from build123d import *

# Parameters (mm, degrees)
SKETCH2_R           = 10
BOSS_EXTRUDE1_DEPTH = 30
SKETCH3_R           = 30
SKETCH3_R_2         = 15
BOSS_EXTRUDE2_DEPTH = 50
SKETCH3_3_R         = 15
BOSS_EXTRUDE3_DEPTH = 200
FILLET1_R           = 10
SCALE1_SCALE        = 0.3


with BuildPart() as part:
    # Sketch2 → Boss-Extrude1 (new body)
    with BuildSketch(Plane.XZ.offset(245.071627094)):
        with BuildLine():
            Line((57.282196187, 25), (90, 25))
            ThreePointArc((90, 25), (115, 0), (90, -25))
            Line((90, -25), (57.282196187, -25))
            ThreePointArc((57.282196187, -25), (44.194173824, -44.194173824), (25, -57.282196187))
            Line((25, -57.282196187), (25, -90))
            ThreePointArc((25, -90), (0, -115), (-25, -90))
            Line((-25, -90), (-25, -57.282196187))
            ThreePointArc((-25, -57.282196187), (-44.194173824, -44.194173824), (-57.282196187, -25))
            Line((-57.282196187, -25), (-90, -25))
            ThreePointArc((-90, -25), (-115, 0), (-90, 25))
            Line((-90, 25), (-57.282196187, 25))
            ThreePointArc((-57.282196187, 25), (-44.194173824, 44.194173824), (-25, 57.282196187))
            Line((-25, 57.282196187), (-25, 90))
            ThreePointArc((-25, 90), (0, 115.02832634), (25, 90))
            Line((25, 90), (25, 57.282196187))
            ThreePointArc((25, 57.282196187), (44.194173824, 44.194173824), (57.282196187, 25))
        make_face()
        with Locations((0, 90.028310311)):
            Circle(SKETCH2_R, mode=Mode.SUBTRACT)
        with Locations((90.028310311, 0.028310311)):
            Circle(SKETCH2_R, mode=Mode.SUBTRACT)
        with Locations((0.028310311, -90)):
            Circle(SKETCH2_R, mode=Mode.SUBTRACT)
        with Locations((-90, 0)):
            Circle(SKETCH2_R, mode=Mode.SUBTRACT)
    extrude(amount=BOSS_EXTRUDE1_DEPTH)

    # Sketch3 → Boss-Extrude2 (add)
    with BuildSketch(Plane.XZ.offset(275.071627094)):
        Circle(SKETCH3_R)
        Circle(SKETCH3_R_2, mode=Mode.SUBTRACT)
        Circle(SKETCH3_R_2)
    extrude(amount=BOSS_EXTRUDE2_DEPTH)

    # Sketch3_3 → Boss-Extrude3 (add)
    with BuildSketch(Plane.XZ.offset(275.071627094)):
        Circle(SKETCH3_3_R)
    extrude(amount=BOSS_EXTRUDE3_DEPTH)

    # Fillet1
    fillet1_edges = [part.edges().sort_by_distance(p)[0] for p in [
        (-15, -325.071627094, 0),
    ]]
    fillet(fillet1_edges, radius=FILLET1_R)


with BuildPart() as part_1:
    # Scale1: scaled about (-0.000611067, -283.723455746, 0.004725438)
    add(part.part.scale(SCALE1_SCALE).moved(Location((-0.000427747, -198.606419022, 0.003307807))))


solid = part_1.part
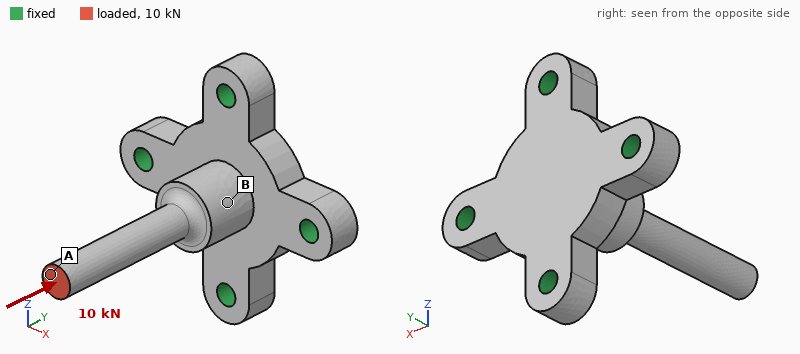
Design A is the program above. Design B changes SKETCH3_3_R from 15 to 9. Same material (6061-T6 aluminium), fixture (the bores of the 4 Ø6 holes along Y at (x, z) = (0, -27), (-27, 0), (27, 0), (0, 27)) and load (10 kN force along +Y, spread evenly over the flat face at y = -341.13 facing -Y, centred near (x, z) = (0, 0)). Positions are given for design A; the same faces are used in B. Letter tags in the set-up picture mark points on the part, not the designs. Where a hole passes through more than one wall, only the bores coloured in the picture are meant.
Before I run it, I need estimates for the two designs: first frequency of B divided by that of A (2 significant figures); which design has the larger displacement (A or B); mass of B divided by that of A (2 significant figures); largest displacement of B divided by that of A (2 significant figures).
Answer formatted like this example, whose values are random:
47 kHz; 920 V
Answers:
0.69; B; 0.92; 2.2
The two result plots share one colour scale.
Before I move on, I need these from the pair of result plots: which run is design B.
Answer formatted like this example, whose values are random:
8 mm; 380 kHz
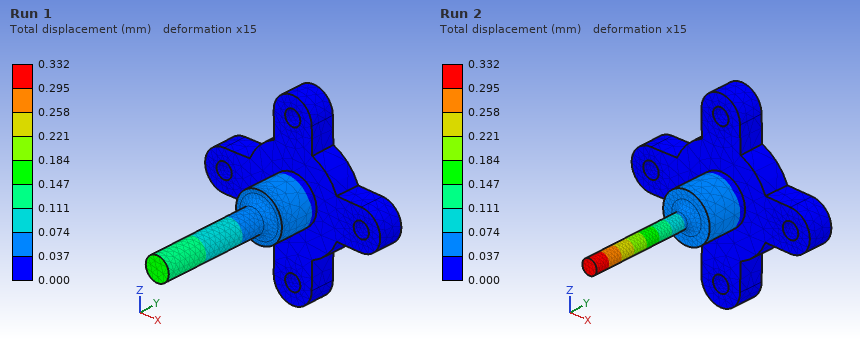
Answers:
Run 2
